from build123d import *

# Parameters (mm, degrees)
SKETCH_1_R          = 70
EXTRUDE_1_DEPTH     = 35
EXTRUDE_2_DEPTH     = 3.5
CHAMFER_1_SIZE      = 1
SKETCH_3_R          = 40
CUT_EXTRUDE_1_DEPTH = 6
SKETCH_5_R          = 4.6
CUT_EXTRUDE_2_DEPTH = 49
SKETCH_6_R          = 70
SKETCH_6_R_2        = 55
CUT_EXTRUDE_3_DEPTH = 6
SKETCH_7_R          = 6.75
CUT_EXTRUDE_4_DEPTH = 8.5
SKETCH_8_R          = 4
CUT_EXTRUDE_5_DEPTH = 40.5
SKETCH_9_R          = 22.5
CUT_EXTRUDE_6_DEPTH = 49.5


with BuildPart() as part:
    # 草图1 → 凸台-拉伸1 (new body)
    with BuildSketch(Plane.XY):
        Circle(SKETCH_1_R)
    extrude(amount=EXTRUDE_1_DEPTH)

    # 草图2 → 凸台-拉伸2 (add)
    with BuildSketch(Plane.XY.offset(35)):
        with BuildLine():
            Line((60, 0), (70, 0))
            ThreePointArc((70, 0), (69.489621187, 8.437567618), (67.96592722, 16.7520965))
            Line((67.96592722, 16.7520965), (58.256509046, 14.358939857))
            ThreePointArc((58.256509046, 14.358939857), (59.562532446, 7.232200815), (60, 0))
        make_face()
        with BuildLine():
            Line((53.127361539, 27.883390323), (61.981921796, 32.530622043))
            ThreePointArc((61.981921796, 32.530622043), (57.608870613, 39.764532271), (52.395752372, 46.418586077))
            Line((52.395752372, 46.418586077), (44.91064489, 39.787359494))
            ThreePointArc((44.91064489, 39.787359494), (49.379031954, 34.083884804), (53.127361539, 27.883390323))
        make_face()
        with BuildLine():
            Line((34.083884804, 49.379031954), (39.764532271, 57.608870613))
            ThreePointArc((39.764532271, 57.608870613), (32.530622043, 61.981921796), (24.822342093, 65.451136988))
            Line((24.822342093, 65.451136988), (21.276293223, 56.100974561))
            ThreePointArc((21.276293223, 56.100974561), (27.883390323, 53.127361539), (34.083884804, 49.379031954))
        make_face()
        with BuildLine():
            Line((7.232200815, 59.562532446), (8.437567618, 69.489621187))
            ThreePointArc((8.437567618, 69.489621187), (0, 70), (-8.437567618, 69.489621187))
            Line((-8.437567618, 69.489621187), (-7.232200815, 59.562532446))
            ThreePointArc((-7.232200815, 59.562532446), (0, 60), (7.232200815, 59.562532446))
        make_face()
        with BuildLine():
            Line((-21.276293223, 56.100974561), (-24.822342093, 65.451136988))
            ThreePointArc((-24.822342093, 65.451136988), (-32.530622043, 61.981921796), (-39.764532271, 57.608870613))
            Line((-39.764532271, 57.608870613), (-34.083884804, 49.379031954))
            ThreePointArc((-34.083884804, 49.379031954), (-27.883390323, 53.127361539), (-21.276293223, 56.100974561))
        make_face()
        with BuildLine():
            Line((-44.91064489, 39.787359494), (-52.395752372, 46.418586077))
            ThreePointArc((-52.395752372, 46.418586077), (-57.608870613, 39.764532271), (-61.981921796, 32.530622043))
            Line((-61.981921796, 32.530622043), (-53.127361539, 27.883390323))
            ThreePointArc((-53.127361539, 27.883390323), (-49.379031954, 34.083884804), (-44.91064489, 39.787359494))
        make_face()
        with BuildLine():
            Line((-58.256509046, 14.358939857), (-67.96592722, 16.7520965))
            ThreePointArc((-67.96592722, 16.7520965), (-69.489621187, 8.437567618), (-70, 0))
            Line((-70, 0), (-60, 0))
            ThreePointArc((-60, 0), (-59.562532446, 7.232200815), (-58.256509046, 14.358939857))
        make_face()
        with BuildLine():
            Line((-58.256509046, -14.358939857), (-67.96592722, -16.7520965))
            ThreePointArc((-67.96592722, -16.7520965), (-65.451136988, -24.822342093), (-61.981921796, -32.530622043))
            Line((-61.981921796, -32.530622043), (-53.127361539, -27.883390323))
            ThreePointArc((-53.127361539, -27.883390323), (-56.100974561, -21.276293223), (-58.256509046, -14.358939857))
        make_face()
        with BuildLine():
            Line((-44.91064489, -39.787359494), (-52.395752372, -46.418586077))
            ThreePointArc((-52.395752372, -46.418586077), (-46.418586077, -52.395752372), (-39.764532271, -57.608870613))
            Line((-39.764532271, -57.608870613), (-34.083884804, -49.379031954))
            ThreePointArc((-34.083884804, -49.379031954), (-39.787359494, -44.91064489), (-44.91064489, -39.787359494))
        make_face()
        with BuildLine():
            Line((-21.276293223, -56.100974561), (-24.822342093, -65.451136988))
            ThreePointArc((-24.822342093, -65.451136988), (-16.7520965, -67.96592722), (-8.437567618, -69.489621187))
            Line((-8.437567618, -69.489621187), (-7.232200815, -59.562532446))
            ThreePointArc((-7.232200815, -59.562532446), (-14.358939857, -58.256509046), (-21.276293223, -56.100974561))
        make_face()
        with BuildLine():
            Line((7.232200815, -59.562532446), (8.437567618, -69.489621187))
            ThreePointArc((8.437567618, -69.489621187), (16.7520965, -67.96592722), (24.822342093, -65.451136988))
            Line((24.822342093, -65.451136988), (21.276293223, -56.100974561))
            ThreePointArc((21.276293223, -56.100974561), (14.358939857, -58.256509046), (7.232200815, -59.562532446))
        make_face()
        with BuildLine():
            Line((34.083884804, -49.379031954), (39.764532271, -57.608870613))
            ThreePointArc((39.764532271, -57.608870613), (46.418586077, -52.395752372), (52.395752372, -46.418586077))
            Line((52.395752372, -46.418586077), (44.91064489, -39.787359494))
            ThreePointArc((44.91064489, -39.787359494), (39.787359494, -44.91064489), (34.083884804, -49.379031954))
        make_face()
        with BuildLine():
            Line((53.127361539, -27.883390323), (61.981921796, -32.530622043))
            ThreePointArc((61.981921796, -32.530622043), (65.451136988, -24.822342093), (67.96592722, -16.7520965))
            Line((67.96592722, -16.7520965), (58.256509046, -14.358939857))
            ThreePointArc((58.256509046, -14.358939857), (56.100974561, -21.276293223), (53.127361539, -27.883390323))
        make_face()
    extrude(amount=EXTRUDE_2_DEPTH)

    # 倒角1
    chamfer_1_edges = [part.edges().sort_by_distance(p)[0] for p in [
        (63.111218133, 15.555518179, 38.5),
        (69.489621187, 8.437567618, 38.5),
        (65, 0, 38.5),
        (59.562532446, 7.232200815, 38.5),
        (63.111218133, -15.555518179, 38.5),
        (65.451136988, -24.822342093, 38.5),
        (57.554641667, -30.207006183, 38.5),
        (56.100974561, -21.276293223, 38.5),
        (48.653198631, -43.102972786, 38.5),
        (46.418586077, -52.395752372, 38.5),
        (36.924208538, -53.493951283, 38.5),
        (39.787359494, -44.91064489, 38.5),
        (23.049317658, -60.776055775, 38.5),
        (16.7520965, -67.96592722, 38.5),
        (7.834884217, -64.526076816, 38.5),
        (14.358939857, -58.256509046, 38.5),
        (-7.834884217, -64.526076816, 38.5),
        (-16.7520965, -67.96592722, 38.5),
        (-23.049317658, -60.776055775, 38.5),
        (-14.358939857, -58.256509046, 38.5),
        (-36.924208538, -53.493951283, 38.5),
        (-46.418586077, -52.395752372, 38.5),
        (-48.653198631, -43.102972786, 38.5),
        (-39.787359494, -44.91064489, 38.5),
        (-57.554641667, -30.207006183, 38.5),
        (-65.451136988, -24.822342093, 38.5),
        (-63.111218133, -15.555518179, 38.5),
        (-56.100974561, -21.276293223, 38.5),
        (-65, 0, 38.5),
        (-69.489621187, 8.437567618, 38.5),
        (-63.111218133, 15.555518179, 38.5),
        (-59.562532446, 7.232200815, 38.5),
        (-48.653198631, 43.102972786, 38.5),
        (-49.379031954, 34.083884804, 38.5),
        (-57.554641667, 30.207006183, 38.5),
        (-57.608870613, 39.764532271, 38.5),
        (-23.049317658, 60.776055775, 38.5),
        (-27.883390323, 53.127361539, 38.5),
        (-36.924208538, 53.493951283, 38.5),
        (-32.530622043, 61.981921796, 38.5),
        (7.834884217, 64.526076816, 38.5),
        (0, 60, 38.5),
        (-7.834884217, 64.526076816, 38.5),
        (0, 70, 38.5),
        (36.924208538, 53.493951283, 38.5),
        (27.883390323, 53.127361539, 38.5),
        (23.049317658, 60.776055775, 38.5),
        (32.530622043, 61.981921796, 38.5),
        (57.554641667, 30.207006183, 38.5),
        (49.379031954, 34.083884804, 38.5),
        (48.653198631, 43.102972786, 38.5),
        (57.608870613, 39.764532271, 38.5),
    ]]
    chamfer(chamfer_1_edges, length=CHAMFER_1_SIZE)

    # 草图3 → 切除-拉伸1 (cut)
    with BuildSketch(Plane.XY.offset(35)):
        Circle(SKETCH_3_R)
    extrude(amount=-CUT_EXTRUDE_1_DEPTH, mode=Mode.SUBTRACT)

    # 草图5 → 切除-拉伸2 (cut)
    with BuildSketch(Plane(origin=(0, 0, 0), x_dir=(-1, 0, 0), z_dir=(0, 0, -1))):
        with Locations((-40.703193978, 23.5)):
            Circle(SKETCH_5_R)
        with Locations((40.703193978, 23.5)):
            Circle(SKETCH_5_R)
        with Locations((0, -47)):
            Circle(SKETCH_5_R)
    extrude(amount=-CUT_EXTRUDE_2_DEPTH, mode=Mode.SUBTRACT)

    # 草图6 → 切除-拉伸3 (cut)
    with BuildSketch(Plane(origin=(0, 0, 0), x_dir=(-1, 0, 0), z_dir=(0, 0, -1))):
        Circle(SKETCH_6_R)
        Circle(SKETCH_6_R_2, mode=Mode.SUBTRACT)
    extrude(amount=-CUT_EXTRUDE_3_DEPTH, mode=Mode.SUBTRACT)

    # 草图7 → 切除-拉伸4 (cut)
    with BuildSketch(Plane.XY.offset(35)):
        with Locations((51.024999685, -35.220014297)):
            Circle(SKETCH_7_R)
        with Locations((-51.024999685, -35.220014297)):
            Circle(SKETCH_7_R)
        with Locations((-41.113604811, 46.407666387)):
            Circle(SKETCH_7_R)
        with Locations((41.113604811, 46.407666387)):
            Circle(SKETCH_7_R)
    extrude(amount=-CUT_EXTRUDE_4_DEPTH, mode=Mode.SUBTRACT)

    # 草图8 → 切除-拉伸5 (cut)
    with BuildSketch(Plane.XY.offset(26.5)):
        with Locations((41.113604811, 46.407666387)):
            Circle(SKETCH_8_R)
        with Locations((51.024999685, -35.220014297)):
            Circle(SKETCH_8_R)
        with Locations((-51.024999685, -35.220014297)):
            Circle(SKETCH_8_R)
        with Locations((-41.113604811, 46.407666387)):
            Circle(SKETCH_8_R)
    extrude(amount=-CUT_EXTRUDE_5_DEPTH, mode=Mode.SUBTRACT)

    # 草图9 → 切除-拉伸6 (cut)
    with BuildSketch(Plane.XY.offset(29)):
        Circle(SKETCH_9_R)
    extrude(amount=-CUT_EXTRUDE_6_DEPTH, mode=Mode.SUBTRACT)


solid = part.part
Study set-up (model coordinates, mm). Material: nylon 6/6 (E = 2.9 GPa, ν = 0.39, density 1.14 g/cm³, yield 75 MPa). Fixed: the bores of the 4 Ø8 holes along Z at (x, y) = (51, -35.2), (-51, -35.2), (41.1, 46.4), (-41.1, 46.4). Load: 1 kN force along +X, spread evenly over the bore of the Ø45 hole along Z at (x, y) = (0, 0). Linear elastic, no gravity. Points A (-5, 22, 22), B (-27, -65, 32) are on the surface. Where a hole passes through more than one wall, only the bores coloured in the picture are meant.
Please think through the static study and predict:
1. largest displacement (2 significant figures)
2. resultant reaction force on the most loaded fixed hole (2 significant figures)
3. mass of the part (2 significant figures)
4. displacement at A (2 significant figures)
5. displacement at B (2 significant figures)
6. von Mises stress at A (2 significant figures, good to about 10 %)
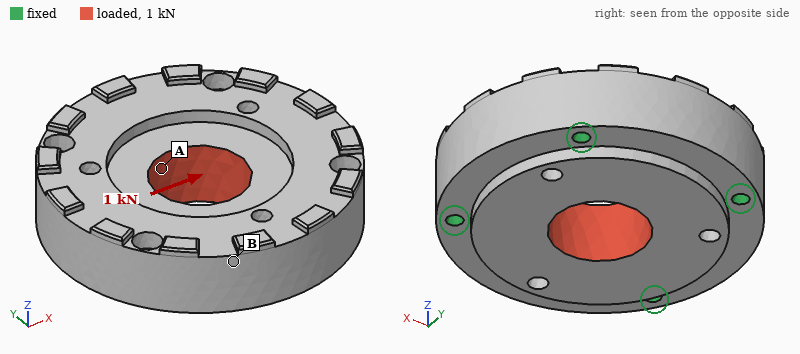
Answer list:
7.5 µm
280 N
480 g
5.5 µm
2.0 µm
0.44 MPa
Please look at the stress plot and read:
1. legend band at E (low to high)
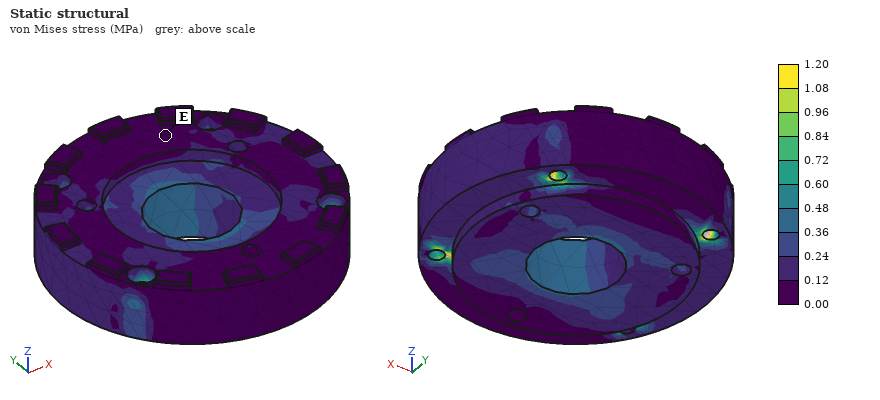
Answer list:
0.00 to 0.12 MPa
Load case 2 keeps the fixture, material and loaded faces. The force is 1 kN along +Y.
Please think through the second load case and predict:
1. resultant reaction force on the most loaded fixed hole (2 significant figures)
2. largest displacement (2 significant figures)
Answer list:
260 N
10 µm
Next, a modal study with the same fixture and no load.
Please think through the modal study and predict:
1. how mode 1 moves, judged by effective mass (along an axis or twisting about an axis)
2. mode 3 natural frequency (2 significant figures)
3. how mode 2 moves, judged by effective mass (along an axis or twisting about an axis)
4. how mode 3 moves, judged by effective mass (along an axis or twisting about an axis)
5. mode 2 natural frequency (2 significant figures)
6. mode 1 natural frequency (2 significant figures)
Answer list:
along Z
3100 Hz
along Z
twisting about X
2800 Hz
2100 Hz
